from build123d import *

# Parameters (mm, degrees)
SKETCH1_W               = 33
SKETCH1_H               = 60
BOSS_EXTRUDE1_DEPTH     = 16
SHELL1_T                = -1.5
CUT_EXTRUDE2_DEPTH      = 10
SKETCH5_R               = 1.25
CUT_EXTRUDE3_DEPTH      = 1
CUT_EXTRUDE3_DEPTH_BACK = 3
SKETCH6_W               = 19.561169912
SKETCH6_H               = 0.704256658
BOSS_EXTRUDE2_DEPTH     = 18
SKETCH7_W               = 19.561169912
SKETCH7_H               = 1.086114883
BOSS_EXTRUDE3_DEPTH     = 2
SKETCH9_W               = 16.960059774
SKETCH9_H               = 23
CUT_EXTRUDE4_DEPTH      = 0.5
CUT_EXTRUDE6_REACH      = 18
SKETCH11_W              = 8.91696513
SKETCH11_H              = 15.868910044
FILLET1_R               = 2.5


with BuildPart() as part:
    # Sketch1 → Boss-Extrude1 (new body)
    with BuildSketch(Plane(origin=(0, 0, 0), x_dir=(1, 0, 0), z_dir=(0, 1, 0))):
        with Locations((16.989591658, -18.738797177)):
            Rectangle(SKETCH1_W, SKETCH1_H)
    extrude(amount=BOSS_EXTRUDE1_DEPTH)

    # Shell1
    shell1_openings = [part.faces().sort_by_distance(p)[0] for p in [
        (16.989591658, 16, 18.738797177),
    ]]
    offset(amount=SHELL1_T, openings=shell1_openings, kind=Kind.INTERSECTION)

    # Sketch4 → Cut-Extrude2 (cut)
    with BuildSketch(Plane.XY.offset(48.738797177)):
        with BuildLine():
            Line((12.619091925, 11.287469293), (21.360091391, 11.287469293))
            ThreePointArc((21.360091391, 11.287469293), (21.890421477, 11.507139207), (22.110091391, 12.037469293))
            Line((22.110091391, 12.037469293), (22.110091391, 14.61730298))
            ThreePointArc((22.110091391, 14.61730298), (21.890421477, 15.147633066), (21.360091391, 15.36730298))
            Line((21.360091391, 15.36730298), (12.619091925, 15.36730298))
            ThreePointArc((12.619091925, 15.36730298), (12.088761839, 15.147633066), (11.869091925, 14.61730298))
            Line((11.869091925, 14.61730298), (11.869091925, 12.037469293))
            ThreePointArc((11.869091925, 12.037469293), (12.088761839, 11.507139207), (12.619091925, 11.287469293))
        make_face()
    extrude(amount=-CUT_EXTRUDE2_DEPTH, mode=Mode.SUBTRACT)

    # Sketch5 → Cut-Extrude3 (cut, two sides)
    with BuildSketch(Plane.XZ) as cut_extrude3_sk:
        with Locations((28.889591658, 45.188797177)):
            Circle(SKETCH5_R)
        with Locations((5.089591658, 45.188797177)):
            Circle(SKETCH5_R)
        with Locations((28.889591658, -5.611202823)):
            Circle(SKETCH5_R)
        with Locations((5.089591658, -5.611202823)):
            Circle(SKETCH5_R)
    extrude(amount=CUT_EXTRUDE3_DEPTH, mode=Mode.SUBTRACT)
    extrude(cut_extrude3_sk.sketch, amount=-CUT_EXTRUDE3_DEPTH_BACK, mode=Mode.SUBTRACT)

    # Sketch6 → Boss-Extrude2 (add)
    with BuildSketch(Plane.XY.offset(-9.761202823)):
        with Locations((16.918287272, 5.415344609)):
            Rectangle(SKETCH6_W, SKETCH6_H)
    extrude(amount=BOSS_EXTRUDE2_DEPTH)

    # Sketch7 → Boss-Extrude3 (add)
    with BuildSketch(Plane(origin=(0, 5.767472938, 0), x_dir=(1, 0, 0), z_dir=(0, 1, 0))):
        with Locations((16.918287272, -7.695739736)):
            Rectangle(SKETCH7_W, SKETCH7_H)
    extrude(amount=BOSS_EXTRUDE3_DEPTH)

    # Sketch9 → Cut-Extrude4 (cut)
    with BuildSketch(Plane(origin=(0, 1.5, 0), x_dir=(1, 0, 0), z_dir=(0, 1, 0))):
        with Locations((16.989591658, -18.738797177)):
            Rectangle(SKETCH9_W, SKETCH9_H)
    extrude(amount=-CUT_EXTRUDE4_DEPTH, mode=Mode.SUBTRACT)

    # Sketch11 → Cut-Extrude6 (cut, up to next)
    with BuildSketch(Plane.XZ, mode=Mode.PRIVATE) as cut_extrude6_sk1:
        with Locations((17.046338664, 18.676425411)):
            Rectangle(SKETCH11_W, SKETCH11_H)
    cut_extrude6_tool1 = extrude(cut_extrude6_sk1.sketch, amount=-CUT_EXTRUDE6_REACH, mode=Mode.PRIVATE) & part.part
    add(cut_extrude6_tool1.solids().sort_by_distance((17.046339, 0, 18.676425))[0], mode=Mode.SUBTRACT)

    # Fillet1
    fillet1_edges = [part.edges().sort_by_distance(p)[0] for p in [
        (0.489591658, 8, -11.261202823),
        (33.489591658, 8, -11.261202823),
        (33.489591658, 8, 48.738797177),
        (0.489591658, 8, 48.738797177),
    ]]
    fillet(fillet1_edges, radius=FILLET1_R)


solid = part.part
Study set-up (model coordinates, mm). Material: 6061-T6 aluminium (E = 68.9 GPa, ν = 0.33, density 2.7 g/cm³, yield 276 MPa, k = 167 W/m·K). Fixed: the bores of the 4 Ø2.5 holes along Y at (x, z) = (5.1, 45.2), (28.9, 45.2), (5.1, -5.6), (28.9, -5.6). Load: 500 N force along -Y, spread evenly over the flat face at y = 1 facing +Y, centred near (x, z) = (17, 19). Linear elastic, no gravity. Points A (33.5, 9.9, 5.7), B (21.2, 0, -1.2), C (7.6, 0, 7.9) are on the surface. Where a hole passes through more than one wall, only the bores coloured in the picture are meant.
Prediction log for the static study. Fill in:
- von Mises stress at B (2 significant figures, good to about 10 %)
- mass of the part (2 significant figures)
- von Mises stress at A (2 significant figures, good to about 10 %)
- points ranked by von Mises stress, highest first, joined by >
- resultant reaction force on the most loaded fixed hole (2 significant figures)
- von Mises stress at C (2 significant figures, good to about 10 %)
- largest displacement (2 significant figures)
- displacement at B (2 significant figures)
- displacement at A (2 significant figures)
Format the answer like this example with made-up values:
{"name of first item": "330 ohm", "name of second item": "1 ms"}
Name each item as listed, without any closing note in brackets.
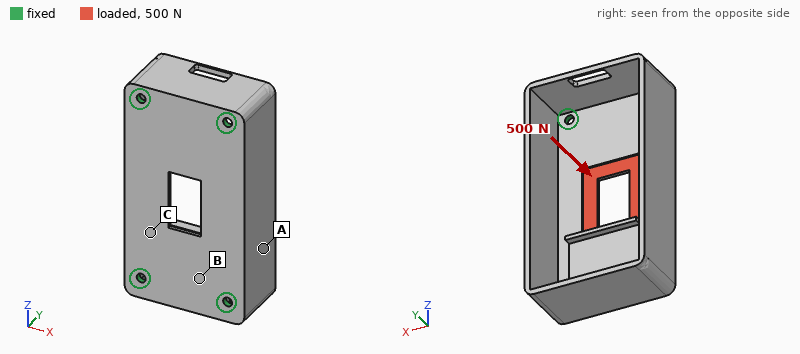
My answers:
{"von Mises stress at B": "60 MPa", "mass of the part": "18 g", "von Mises stress at A": "28 MPa", "points ranked by von Mises stress, highest first, joined by >": "C > B > A", "resultant reaction force on the most loaded fixed hole": "140 N", "von Mises stress at C": "94 MPa", "largest displacement": "0.30 mm", "displacement at B": "0.046 mm", "displacement at A": "0.088 mm"}
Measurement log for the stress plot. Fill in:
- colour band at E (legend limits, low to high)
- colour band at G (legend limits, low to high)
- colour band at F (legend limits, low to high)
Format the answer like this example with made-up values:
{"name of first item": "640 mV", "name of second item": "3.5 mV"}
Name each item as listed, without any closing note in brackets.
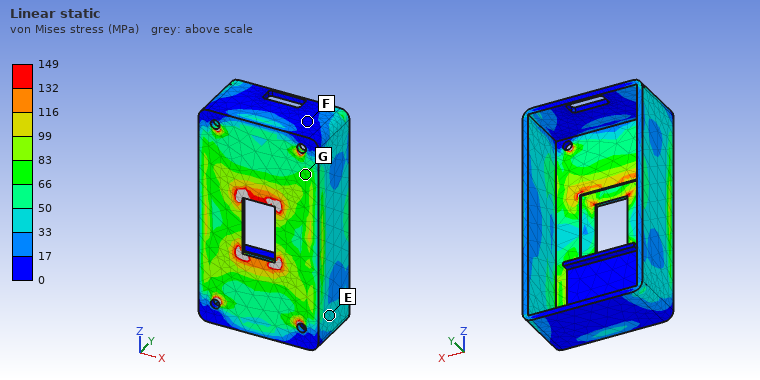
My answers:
{"colour band at E": "33 to 50 MPa", "colour band at G": "66 to 83 MPa", "colour band at F": "0 to 17 MPa"}
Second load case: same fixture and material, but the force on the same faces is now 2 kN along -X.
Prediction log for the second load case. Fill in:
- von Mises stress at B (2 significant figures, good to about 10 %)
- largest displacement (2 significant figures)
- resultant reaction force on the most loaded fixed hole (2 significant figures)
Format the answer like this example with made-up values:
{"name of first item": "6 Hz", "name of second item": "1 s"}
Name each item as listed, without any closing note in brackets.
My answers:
{"von Mises stress at B": "42 MPa", "largest displacement": "31 µm", "resultant reaction force on the most loaded fixed hole": "630 N"}
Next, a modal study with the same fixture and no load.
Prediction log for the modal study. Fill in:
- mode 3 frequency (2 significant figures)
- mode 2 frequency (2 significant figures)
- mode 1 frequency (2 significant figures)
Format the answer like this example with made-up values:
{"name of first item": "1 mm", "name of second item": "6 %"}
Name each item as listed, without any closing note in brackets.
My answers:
{"mode 3 frequency": "3900 Hz", "mode 2 frequency": "3500 Hz", "mode 1 frequency": "1400 Hz"}
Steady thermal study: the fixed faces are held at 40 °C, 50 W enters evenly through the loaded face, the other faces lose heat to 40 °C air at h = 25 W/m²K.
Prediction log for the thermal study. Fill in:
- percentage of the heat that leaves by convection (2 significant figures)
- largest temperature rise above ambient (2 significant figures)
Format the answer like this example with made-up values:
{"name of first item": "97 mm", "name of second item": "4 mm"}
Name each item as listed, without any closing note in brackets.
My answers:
{"percentage of the heat that leaves by convection": "9.3 %", "largest temperature rise above ambient": "58 K"}
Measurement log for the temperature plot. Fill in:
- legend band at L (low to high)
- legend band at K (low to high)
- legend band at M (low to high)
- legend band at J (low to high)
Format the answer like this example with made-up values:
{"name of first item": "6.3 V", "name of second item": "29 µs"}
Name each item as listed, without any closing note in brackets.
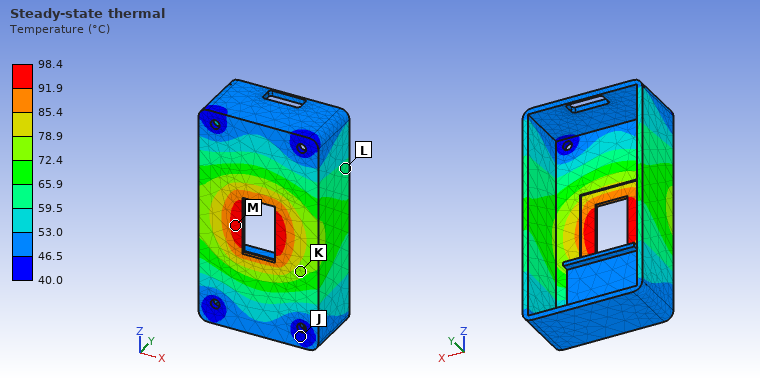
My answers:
{"legend band at L": "59.5 to 65.9 °C", "legend band at K": "72.4 to 78.9 °C", "legend band at M": "91.9 to 98.4 °C", "legend band at J": "40.0 to 46.5 °C"}
